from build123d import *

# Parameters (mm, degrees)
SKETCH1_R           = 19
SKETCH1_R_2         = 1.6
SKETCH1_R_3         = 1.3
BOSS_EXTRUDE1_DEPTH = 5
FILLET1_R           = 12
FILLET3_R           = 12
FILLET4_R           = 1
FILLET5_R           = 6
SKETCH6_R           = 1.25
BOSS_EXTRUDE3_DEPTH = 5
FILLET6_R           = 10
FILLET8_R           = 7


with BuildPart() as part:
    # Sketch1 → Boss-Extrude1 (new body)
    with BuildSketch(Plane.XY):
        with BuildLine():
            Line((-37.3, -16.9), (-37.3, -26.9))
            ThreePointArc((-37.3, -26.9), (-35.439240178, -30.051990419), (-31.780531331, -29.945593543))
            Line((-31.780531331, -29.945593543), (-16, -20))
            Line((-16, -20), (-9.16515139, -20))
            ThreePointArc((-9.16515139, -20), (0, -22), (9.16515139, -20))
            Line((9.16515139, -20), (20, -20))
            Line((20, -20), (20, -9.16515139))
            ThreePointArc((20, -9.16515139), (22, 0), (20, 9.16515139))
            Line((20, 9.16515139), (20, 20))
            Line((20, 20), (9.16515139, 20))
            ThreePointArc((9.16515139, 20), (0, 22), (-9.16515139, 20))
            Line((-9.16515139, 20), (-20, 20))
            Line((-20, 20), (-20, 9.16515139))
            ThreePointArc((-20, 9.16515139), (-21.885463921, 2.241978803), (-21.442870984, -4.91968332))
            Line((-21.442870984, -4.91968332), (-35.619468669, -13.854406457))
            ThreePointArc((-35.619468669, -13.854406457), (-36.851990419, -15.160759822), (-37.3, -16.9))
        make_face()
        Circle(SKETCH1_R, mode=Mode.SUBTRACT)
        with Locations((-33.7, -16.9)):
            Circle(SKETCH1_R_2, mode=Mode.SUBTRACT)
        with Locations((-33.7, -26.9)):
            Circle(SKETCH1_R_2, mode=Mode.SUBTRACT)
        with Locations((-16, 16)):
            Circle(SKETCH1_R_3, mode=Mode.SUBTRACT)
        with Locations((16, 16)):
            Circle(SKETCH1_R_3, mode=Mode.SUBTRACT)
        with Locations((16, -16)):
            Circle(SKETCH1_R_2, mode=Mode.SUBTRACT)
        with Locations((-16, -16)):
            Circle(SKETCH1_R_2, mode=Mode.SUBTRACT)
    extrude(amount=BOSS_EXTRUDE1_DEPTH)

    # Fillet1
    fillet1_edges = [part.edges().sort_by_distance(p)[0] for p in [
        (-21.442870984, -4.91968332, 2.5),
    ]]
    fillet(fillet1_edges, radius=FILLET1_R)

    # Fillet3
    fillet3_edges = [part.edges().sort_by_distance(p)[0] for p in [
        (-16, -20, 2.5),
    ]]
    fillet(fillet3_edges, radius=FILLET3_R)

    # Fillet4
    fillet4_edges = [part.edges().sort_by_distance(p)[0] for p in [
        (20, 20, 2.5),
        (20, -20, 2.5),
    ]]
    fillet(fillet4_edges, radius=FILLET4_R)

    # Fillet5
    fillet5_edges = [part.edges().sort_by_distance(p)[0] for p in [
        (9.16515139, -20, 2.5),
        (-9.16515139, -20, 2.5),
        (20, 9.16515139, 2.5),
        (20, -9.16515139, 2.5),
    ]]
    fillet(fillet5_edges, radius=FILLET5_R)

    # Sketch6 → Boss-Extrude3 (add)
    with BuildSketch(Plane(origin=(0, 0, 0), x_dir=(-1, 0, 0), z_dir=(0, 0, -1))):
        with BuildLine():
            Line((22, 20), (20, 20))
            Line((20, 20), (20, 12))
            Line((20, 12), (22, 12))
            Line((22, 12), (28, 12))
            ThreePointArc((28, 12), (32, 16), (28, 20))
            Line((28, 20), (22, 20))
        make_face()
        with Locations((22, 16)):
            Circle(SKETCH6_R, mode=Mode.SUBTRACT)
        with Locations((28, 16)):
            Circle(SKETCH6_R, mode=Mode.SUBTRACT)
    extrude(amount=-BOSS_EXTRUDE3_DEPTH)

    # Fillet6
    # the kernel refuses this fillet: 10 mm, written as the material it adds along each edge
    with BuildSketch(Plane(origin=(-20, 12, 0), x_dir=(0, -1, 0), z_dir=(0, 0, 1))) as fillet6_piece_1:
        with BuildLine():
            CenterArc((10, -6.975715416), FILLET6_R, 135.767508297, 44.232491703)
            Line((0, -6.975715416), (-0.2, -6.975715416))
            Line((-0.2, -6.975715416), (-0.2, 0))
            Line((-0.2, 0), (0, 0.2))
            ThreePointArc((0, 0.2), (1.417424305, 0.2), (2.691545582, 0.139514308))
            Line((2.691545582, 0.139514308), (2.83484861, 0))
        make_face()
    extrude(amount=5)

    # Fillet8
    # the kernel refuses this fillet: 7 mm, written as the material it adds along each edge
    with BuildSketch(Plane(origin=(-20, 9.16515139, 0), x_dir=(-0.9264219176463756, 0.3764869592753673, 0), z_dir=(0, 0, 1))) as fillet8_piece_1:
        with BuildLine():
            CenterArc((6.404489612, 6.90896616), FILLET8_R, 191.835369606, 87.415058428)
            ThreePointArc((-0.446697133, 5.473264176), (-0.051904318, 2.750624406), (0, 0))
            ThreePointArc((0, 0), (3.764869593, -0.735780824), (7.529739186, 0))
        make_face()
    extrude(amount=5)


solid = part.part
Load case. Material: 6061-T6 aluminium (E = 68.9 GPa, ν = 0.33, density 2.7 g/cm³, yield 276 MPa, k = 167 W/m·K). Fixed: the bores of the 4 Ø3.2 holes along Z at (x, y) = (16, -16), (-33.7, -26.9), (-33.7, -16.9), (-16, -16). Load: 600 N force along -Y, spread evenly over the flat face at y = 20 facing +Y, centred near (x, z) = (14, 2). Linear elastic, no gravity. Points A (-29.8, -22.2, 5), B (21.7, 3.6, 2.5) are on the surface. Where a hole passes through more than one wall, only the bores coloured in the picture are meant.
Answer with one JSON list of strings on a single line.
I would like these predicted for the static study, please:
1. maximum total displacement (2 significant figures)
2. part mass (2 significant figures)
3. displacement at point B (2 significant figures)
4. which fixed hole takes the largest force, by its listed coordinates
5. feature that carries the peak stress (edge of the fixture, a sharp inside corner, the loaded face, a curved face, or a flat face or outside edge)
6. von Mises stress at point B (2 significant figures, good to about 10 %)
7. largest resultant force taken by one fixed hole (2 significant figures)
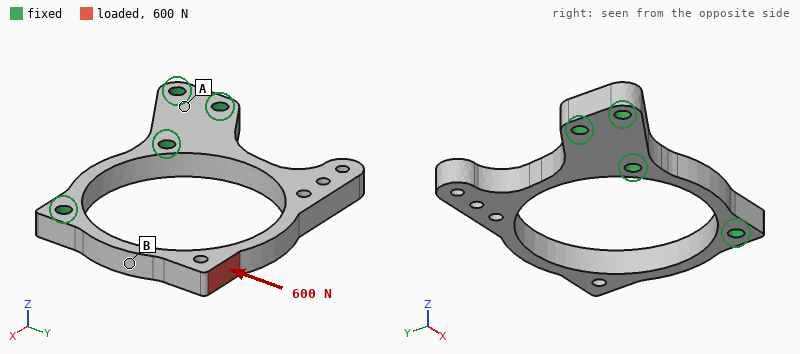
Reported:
["80 µm", "13 g", "73 µm", "(16, -16)", "a curved face", "68 MPa", "540 N"]
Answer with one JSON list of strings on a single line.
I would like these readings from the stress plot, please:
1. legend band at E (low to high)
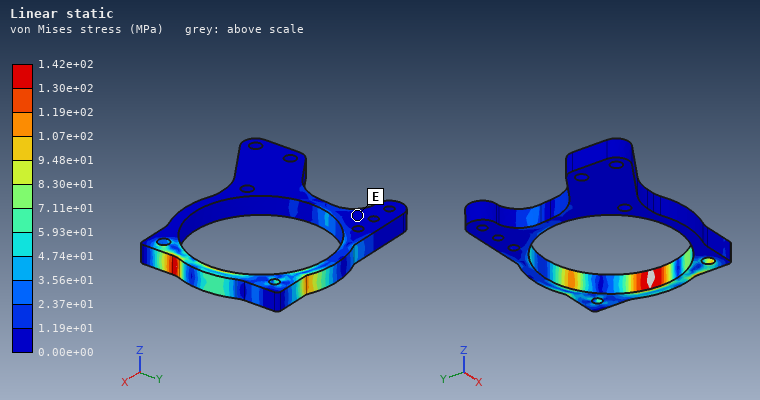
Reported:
["0.00e+00 to 1.19e+01 MPa"]
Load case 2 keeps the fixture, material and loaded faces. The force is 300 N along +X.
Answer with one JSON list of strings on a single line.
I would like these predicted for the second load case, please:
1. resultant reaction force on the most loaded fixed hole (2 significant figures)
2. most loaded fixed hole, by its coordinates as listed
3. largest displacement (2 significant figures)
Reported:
["240 N", "(-33.7, -16.9)", "0.19 mm"]
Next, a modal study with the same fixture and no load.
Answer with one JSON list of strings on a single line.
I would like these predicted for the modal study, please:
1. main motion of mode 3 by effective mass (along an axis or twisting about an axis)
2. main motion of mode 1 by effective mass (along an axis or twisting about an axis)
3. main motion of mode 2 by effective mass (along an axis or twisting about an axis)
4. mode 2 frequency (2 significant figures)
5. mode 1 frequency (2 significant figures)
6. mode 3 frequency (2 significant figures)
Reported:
["along X", "along Z", "twisting about Y", "3100 Hz", "1900 Hz", "3300 Hz"]
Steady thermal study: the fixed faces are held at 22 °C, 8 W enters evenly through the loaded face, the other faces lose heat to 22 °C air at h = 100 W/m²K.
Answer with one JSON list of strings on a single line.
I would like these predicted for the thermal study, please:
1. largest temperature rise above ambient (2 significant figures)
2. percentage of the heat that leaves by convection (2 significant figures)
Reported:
["41 K", "43 %"]
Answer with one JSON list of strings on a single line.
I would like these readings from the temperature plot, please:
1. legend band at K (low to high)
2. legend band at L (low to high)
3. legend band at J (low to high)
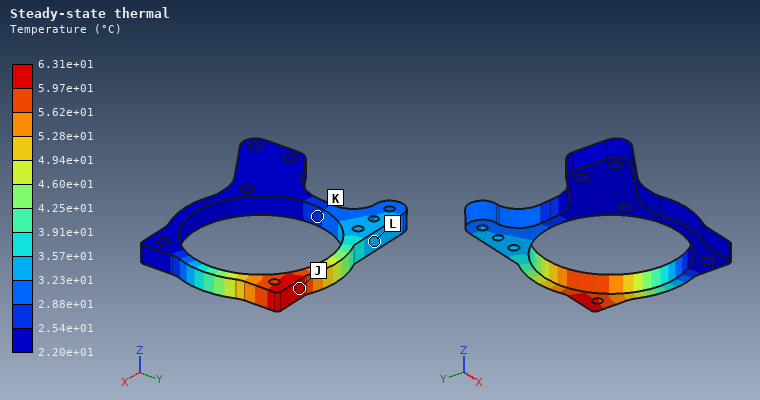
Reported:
["2.54e+01 to 2.88e+01 °C", "3.23e+01 to 3.57e+01 °C", "5.97e+01 to 6.31e+01 °C"]
